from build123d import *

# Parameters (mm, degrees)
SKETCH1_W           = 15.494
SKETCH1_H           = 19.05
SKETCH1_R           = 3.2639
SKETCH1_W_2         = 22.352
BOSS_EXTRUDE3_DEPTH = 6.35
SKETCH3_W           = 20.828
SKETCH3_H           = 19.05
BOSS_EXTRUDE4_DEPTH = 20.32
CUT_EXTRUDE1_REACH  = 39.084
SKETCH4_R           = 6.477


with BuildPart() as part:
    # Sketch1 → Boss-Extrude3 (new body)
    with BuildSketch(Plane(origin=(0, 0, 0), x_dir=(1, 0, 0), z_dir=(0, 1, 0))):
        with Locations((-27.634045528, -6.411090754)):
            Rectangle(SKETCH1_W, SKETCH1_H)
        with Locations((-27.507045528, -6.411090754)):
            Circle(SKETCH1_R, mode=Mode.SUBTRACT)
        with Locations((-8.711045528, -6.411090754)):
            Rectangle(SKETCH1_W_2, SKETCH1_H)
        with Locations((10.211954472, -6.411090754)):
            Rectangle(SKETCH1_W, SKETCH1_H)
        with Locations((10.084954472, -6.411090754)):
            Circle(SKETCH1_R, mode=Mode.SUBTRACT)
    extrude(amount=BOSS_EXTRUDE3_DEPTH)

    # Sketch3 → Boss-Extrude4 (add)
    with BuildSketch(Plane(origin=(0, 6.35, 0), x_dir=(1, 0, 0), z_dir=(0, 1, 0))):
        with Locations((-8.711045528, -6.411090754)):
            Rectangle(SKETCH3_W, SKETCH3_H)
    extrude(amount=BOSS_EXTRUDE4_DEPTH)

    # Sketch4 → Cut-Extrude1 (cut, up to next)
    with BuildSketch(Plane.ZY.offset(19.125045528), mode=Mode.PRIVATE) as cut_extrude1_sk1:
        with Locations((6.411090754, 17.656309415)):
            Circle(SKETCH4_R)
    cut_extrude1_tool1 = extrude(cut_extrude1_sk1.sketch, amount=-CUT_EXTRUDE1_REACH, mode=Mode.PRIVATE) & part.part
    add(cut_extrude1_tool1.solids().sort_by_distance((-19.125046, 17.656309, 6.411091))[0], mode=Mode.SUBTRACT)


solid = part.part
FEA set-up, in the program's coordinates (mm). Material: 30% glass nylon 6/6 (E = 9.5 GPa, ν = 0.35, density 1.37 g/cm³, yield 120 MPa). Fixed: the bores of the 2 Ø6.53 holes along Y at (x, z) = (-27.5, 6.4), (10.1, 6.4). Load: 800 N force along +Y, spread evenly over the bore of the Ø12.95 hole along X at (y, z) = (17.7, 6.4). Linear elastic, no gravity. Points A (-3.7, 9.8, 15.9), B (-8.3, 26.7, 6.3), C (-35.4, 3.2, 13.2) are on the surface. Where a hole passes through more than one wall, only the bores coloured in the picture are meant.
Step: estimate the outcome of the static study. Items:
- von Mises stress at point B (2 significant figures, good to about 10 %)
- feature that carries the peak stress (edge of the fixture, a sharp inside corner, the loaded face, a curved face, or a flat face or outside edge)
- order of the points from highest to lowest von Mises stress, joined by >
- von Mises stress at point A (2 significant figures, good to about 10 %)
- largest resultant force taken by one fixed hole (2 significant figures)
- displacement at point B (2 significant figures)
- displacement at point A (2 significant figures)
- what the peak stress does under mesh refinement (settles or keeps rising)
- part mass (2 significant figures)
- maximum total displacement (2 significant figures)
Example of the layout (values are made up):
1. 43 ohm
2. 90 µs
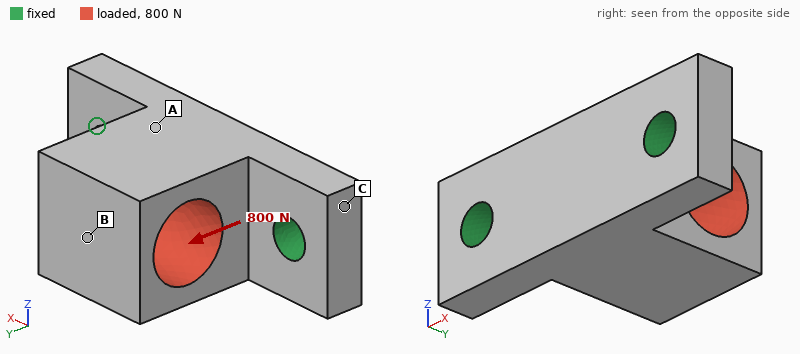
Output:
1. 7.7 MPa
2. edge of the fixture
3. B > A > C
4. 4.4 MPa
5. 430 N
6. 37 µm
7. 24 µm
8. keeps rising
9. 16 g
10. 38 µm
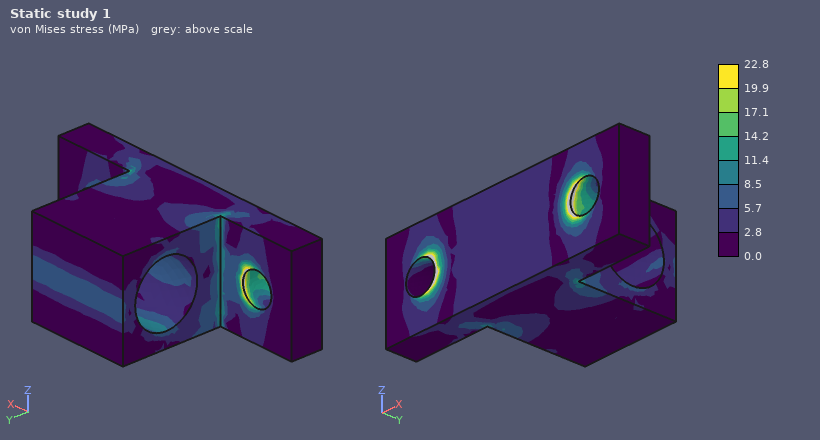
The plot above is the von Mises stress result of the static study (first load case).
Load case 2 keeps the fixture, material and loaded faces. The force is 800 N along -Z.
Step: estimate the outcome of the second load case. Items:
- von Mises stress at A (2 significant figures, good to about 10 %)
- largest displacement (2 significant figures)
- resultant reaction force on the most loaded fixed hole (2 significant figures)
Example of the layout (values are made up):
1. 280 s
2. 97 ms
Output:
1. 11 MPa
2. 0.30 mm
3. 400 N
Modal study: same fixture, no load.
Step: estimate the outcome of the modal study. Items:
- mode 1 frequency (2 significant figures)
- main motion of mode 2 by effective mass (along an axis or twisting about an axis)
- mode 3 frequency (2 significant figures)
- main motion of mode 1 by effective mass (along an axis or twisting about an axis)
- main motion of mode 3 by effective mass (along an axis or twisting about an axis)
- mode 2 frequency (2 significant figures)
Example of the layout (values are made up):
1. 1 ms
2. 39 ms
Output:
1. 3700 Hz
2. along X
3. 8900 Hz
4. along Z
5. along Y
6. 7800 Hz
